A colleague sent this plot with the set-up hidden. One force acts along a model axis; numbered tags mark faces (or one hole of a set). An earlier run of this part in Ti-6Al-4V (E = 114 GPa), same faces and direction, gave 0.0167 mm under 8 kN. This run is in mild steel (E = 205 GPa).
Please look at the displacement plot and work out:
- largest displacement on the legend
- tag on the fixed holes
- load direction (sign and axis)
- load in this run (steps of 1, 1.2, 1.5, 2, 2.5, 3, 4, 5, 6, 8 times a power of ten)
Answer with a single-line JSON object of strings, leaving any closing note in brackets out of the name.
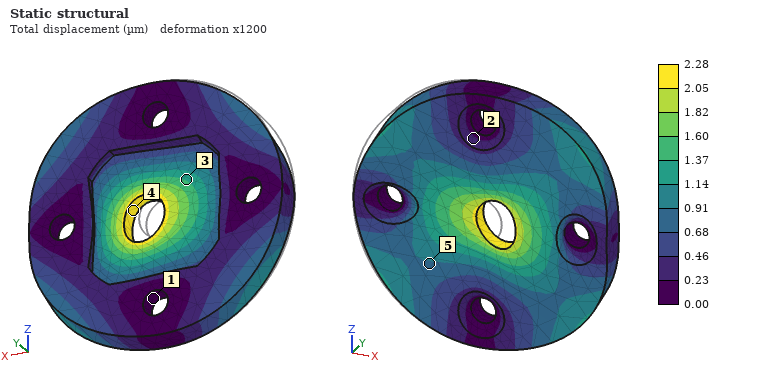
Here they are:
{"largest displacement on the legend": "2.28 µm", "tag on the fixed holes": "1", "load direction": "+X", "load in this run": "2 kN"}
